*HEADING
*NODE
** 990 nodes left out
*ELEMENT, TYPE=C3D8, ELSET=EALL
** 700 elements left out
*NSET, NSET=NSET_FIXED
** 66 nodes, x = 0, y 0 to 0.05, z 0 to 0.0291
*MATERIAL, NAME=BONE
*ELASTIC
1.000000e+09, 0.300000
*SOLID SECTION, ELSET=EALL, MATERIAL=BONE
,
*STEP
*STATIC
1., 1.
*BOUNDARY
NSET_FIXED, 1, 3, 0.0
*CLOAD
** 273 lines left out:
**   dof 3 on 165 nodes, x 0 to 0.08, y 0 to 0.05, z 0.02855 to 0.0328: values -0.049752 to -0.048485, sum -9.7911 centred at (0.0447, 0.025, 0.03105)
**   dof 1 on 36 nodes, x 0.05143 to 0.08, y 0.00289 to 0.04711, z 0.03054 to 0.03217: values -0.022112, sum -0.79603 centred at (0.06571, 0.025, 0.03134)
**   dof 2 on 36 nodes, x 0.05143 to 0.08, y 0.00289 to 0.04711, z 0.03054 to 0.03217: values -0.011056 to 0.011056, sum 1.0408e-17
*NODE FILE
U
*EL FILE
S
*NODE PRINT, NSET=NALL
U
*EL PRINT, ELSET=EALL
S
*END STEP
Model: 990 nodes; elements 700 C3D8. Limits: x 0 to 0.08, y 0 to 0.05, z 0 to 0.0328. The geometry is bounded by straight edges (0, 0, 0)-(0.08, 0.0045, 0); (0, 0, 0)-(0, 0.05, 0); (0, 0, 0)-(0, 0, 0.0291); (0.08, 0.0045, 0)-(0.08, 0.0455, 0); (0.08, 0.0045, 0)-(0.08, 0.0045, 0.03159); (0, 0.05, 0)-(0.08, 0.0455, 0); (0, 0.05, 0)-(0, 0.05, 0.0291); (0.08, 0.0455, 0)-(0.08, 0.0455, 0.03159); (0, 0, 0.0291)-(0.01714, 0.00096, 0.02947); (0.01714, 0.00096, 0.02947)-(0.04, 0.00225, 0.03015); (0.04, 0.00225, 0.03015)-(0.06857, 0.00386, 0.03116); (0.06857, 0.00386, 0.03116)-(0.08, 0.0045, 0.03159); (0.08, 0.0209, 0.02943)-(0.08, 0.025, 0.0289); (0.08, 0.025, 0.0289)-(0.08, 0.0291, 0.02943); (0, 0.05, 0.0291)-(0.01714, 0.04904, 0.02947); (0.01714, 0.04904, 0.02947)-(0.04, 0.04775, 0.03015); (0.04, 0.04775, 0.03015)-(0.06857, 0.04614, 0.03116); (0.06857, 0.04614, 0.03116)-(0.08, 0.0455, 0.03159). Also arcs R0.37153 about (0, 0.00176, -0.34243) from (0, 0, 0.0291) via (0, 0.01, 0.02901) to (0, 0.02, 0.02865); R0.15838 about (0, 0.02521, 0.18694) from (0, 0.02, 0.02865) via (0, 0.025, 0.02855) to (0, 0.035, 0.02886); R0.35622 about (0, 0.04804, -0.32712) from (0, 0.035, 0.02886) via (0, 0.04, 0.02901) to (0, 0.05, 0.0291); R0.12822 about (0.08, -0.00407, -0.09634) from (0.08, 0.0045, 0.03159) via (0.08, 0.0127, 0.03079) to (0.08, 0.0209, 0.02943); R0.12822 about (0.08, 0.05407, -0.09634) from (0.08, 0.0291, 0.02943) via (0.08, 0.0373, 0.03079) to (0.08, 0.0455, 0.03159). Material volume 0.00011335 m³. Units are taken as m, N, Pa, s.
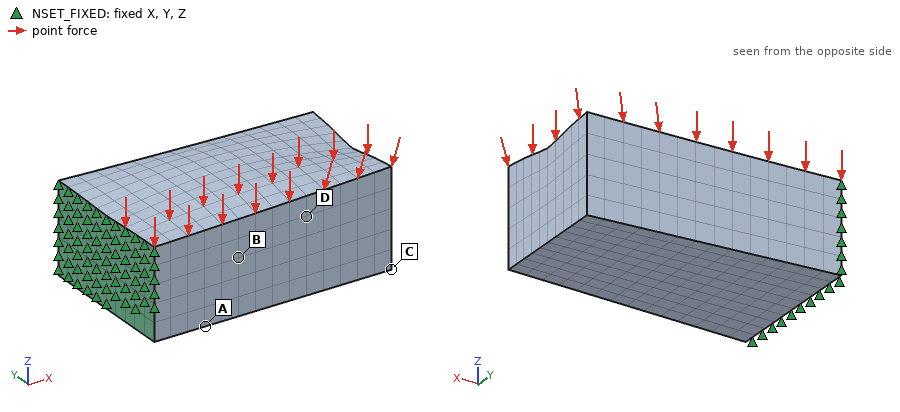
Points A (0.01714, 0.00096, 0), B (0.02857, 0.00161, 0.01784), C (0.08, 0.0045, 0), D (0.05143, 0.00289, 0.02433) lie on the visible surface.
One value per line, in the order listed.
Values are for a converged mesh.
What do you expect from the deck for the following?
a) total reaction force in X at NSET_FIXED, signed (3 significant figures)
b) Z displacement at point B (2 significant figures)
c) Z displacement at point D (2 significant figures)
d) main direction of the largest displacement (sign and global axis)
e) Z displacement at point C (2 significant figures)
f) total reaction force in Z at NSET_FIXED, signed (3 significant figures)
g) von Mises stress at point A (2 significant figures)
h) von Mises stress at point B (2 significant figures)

0.796 N
-1.6e-06 m
-4.1e-06 m
-Z
-7.2e-06 m
9.79 N
36000 Pa
16000 Pa
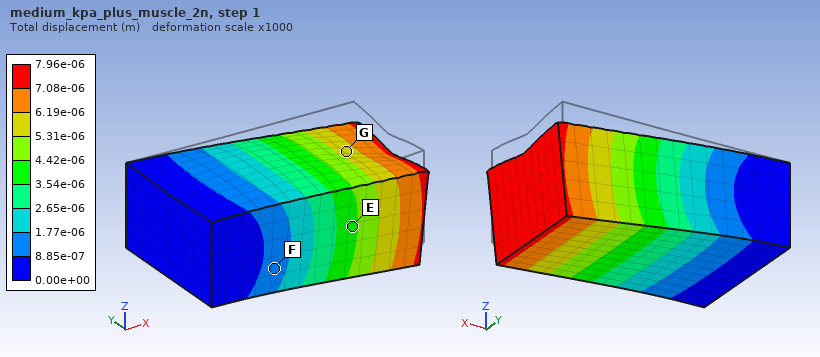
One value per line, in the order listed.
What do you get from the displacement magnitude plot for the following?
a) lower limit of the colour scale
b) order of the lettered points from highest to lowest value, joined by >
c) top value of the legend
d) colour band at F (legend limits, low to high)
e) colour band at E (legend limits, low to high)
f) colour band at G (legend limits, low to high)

0.00e+00 m
G > E > F
7.96e-06 m
8.85e-07 to 1.77e-06 m
3.54e-06 to 4.42e-06 m
5.31e-06 to 6.19e-06 m
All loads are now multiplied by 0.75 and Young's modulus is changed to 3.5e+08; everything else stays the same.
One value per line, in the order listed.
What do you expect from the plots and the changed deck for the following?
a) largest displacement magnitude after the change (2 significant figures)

1.7e-05 m
